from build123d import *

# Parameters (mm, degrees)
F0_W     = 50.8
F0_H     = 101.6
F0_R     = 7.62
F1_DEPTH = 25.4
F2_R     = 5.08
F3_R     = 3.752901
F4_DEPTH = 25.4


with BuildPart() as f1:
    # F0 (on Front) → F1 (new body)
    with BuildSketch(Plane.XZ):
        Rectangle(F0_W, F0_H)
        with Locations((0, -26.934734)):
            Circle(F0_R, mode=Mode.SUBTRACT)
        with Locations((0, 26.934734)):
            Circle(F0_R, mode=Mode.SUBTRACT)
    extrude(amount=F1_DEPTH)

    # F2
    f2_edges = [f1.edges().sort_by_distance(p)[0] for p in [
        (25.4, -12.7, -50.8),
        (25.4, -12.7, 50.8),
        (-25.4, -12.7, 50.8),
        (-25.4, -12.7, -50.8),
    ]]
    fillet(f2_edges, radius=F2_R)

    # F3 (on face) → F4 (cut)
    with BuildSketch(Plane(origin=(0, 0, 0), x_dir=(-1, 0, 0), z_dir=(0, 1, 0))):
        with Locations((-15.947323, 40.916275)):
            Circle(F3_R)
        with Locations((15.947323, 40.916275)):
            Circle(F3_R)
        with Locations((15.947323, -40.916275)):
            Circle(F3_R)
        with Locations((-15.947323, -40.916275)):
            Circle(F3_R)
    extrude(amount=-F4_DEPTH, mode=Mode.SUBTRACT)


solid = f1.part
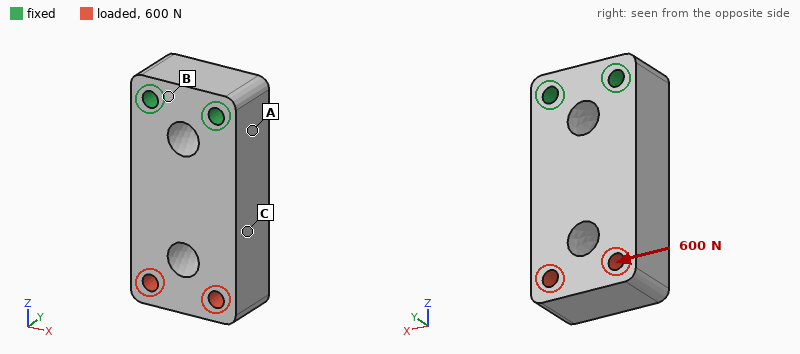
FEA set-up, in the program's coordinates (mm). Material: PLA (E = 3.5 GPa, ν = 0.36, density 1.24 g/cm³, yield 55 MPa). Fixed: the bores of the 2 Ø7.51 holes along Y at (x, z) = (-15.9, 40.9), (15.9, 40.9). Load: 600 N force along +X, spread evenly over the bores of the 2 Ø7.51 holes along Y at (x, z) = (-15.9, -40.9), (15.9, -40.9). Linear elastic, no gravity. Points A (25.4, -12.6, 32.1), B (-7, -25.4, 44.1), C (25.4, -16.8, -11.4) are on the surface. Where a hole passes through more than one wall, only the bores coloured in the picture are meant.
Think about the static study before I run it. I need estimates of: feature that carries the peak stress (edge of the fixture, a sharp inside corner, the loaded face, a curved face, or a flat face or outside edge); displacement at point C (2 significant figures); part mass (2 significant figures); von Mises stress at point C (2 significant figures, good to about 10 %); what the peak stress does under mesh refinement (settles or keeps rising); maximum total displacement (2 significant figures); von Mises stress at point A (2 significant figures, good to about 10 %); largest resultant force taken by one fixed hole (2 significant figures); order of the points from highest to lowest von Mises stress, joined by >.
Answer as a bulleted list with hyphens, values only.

- edge of the fixture
- 0.10 mm
- 140 g
- 2.1 MPa
- keeps rising
- 0.20 mm
- 3.4 MPa
- 1.3 kN
- A > C > B
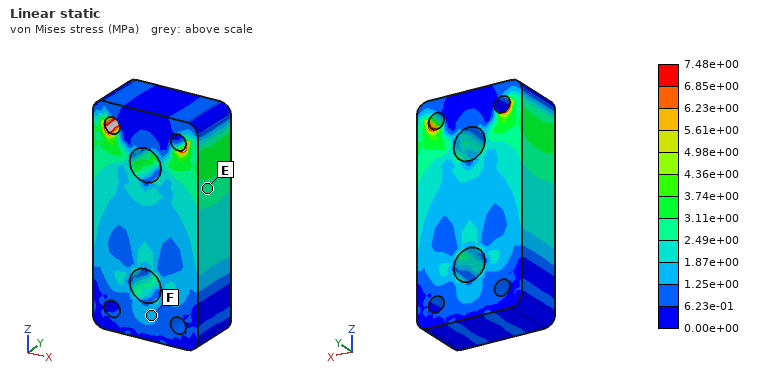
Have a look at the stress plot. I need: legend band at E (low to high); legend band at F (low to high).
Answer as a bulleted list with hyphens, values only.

- 2.49e+00 to 3.11e+00 MPa
- 1.25e+00 to 1.87e+00 MPa
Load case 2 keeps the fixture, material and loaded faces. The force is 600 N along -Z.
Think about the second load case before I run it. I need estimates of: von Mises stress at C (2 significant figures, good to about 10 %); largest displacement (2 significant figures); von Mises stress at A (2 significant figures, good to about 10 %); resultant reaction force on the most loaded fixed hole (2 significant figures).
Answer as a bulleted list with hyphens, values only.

- 0.60 MPa
- 16 µm
- 0.37 MPa
- 300 N
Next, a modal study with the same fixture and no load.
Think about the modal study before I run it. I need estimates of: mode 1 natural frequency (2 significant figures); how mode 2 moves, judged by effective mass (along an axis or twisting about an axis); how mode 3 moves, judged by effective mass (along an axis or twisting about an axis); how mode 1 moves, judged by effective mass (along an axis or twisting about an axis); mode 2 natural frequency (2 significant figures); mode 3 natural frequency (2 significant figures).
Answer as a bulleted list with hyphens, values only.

- 750 Hz
- along X
- twisting about Z
- along Y
- 1300 Hz
- 2100 Hz
